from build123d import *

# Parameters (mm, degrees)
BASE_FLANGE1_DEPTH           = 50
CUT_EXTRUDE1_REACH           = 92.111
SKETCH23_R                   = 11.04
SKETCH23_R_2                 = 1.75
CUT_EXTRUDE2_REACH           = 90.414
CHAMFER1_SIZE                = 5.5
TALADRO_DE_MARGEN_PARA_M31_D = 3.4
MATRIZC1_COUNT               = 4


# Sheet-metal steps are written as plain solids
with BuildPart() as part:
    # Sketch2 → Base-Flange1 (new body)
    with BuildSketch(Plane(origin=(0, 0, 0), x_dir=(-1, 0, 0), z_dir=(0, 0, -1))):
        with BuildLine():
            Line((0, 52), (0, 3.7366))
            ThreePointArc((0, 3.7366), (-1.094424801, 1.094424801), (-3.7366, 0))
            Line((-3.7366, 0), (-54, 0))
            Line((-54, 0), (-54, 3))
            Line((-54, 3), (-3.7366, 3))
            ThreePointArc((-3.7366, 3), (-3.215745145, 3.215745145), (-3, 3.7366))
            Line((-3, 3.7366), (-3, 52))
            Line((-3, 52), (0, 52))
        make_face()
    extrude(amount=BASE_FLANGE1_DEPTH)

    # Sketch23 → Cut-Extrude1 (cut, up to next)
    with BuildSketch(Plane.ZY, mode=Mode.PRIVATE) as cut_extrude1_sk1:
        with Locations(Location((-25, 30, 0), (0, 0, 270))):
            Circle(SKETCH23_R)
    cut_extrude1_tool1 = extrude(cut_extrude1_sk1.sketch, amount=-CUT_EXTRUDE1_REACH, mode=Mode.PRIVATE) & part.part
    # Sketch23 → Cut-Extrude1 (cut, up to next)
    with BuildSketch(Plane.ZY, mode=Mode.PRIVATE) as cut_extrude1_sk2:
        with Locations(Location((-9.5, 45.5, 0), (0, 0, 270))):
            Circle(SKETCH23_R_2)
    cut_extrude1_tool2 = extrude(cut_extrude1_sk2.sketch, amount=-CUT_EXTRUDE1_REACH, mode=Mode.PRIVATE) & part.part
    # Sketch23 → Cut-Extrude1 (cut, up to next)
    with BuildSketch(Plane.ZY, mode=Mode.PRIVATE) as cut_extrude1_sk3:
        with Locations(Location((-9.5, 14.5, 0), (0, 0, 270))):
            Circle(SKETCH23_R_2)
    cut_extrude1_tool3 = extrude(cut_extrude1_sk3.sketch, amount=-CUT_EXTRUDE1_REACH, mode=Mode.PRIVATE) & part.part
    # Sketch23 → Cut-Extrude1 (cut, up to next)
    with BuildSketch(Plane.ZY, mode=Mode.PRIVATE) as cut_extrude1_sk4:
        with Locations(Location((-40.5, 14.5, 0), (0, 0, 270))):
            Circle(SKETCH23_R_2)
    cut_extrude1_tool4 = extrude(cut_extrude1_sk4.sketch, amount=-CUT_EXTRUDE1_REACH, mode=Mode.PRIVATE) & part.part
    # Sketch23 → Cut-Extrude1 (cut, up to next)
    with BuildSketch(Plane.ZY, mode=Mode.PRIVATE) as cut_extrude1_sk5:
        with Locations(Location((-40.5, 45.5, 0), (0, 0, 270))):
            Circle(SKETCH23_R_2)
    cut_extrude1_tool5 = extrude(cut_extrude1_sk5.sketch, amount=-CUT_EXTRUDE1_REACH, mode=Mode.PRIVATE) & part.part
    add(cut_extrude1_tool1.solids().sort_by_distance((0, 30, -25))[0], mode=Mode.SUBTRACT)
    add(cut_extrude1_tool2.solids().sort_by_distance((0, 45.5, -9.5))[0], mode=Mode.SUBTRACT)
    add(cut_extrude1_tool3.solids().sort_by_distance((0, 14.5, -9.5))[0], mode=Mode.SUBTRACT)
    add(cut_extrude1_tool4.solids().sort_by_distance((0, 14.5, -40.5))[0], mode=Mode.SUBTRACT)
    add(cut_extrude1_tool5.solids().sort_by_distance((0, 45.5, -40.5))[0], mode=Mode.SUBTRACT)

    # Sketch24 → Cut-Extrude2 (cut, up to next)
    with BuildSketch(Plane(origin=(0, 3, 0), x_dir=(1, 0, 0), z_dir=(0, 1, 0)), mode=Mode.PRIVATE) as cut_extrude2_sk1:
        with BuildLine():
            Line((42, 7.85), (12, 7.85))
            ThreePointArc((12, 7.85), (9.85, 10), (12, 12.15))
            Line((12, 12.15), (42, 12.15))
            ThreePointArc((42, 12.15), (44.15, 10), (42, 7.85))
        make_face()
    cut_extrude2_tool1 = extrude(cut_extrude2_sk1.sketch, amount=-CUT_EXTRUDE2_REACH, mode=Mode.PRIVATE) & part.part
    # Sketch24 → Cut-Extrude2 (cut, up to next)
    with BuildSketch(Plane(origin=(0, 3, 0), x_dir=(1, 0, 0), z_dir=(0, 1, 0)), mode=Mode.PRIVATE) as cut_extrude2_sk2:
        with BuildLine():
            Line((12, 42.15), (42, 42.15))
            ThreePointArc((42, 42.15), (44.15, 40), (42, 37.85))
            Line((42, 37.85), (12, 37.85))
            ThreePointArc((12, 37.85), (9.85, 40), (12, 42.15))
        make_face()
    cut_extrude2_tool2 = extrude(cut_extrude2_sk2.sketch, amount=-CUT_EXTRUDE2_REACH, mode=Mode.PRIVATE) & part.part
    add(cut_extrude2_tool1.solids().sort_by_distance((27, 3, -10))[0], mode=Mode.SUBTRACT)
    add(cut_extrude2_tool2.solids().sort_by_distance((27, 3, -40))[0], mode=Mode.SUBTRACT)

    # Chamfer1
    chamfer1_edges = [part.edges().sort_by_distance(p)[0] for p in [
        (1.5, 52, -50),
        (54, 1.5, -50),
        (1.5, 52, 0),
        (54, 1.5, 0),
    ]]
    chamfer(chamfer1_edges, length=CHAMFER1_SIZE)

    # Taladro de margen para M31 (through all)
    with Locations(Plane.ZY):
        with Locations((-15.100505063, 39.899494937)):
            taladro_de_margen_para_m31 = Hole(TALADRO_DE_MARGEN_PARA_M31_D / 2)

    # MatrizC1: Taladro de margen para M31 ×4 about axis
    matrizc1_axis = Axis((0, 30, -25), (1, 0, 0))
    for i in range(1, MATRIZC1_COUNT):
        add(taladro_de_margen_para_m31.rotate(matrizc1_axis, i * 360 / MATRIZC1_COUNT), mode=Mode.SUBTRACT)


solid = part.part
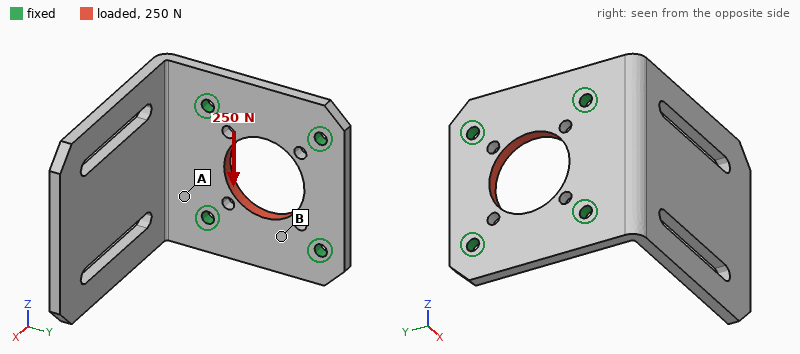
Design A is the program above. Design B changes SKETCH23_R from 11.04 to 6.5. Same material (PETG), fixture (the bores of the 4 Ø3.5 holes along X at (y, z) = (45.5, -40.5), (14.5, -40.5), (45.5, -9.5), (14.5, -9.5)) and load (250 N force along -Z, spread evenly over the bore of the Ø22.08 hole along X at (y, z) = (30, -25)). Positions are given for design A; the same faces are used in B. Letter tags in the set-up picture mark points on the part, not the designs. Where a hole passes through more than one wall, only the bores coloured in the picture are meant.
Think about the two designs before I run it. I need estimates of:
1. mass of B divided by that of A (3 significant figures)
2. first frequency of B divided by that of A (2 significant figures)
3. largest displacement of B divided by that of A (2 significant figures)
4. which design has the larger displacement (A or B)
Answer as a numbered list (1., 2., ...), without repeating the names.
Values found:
1. 1.06
2. 1.0
3. 1.1
4. B
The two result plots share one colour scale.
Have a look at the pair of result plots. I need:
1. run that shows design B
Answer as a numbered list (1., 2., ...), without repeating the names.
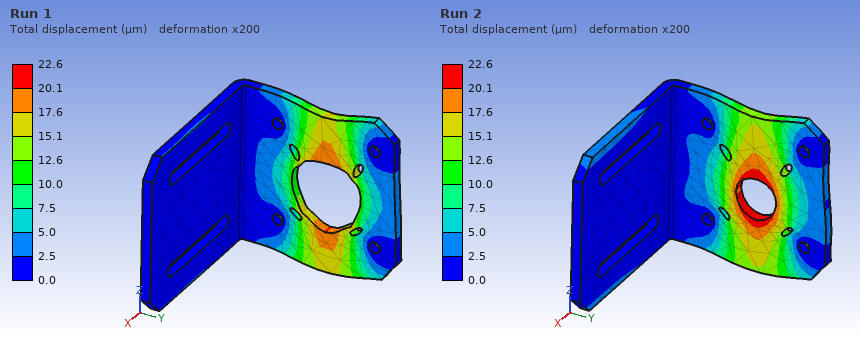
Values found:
1. Run 2
